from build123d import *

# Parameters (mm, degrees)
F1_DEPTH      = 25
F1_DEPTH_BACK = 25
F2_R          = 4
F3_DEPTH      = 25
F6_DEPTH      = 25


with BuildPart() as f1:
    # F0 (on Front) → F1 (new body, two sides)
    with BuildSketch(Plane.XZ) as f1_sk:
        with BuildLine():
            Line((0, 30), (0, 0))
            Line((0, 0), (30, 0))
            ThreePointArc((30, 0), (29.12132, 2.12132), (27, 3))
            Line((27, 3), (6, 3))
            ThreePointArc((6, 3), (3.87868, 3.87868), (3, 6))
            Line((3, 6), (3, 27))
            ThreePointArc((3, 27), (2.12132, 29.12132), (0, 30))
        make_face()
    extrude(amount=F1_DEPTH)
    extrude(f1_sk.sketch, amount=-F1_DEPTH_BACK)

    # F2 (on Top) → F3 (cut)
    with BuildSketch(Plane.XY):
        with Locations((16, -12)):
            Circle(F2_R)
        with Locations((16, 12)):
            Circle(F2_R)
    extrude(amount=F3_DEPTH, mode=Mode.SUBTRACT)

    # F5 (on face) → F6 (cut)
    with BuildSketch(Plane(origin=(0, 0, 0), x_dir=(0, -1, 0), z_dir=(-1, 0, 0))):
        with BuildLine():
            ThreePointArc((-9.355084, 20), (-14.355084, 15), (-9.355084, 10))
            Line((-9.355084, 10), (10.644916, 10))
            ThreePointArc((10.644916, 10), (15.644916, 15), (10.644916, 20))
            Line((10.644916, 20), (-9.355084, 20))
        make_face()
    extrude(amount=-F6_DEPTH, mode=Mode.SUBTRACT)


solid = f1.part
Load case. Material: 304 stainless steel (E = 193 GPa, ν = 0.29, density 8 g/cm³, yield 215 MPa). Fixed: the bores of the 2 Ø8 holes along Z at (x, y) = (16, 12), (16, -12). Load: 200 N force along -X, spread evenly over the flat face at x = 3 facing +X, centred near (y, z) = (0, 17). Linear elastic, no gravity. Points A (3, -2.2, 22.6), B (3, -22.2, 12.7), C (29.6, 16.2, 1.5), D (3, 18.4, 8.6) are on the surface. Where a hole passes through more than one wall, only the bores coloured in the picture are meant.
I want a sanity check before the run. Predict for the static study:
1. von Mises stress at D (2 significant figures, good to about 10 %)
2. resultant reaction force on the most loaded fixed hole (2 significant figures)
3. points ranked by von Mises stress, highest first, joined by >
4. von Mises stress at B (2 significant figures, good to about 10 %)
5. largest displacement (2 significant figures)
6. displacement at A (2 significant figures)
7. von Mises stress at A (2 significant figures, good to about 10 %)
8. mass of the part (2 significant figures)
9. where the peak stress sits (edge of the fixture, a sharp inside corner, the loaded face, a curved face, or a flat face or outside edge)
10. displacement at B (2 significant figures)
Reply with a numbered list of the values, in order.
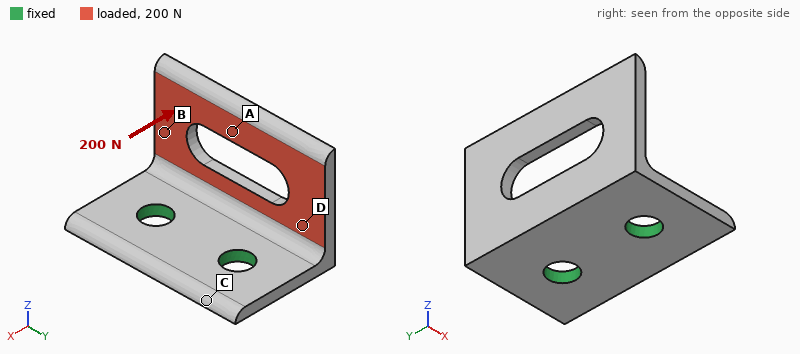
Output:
1. 41 MPa
2. 100 N
3. D > B > A > C
4. 34 MPa
5. 87 µm
6. 60 µm
7. 9.3 MPa
8. 59 g
9. a flat face or outside edge
10. 24 µm
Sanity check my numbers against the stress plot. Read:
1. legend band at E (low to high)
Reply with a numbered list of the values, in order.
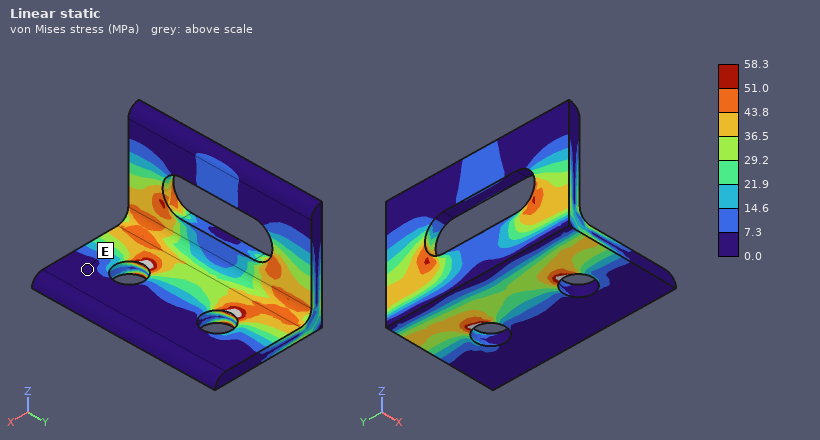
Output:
1. 0.0 to 7.3 MPa
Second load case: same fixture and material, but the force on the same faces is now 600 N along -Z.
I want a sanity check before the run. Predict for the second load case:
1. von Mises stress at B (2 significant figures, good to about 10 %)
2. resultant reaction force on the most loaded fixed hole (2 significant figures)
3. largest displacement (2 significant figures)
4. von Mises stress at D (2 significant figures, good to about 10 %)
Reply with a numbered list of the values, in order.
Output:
1. 18 MPa
2. 310 N
3. 30 µm
4. 25 MPa
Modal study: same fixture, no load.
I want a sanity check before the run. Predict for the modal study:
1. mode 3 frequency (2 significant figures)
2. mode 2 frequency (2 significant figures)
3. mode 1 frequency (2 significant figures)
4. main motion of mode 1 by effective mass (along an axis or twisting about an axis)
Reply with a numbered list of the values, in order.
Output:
1. 5400 Hz
2. 3400 Hz
3. 1800 Hz
4. along X
